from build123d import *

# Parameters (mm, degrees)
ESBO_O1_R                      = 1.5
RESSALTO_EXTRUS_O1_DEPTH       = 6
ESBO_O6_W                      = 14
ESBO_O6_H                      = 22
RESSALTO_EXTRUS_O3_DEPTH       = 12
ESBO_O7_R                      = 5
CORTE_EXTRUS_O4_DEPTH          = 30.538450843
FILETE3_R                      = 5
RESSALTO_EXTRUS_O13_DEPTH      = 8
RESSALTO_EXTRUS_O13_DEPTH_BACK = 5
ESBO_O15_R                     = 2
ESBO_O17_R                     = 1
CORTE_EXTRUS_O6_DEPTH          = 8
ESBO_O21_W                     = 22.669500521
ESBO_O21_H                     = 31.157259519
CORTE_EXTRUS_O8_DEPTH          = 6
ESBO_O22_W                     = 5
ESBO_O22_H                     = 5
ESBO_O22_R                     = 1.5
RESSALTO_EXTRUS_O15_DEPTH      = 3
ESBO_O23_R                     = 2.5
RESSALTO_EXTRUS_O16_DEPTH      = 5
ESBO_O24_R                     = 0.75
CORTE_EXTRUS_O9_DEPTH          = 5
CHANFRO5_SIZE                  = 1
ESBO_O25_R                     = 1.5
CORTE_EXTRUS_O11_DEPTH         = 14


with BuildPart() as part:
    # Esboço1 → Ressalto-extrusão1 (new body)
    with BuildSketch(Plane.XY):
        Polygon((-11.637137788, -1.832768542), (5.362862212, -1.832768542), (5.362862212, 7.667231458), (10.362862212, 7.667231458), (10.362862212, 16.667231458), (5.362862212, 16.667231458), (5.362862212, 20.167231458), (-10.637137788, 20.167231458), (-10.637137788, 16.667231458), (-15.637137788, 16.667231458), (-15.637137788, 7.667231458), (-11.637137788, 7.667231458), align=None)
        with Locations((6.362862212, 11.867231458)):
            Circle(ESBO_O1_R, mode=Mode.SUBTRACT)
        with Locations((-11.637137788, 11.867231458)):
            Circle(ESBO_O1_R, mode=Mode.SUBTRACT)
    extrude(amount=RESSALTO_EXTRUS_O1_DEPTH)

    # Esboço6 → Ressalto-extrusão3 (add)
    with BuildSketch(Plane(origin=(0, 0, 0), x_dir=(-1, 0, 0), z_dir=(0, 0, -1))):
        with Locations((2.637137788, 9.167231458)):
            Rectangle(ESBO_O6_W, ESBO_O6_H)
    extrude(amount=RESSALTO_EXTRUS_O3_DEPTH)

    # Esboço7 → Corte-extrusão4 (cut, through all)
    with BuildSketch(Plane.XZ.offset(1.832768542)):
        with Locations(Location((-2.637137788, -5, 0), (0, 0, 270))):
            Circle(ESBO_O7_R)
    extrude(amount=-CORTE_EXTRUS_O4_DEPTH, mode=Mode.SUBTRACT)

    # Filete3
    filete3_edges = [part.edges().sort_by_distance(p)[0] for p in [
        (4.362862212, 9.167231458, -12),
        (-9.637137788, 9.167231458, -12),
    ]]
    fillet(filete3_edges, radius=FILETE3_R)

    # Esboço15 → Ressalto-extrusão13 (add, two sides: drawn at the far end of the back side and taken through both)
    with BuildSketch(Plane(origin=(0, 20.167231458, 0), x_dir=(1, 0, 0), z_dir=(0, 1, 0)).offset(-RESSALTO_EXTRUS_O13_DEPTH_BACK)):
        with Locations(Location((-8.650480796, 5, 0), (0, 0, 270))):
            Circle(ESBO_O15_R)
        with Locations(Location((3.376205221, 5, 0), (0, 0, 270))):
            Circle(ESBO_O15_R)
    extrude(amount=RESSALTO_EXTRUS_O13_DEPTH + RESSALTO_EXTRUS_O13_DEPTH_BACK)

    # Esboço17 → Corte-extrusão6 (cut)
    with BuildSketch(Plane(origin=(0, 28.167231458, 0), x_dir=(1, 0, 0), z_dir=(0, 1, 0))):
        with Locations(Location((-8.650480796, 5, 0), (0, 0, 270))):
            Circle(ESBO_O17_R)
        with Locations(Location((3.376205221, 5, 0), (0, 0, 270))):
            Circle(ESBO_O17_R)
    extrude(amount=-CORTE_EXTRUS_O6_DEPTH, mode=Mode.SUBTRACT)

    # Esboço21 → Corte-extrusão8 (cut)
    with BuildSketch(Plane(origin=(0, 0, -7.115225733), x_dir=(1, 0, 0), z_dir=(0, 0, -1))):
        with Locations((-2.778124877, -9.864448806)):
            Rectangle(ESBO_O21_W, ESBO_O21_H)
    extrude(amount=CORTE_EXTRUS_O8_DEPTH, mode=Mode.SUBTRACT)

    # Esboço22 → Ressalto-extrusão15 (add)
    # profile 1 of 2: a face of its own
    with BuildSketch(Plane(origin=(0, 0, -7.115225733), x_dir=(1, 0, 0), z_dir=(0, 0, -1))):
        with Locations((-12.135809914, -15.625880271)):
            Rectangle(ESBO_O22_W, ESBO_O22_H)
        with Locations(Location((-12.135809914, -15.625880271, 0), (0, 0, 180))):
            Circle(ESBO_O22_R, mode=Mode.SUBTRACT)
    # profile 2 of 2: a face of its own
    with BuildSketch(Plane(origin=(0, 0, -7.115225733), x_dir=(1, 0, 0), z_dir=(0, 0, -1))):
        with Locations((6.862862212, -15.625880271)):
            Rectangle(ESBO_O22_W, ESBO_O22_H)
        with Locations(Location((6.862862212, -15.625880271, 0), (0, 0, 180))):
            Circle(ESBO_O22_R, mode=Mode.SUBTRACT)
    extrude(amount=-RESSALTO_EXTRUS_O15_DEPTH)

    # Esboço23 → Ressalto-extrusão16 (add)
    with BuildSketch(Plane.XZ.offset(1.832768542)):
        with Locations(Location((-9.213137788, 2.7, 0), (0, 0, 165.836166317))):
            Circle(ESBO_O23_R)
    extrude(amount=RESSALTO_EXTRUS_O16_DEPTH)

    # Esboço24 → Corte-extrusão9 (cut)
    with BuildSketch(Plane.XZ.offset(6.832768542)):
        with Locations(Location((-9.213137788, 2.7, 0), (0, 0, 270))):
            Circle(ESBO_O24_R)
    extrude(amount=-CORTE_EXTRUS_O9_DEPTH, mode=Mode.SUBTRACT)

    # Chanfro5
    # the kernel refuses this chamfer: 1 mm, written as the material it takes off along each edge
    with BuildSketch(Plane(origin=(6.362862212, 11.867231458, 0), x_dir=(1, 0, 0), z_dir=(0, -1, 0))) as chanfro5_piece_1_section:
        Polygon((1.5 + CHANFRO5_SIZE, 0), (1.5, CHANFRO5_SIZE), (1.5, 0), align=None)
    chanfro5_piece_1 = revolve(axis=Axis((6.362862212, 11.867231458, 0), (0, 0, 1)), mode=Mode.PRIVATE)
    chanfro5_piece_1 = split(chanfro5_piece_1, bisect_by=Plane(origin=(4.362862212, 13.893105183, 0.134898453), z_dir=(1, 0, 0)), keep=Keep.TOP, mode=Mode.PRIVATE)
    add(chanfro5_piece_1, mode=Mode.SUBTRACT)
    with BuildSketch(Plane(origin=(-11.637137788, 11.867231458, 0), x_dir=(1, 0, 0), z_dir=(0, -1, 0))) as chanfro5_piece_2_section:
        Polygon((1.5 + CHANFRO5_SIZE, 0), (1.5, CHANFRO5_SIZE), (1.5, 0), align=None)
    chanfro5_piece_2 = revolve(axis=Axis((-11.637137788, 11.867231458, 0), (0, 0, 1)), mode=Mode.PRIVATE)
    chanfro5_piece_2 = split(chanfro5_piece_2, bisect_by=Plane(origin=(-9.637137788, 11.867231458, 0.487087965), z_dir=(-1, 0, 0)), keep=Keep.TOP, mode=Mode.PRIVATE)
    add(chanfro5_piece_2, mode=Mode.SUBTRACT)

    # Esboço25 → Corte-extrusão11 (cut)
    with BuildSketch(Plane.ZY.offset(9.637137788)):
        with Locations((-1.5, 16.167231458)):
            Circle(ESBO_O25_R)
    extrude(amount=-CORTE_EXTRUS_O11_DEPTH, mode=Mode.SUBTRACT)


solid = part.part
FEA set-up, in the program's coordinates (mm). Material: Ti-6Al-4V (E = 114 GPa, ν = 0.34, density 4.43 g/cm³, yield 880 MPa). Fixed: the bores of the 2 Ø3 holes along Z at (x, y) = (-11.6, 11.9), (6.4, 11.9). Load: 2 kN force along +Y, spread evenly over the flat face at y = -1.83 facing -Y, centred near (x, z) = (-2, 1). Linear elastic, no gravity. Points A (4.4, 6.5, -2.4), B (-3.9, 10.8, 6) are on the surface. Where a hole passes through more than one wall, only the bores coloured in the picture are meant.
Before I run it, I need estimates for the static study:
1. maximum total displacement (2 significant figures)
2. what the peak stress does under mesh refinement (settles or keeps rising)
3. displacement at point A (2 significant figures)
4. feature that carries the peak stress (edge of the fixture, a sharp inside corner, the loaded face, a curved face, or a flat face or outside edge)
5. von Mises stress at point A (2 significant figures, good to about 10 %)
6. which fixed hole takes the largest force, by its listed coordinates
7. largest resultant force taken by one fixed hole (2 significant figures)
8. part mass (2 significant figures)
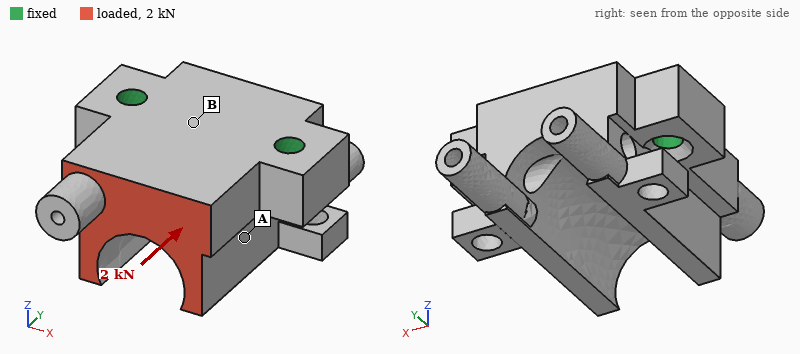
11 µm
keeps rising
5.4 µm
edge of the fixture
19 MPa
(6.4, 11.9)
1.1 kN
17 g
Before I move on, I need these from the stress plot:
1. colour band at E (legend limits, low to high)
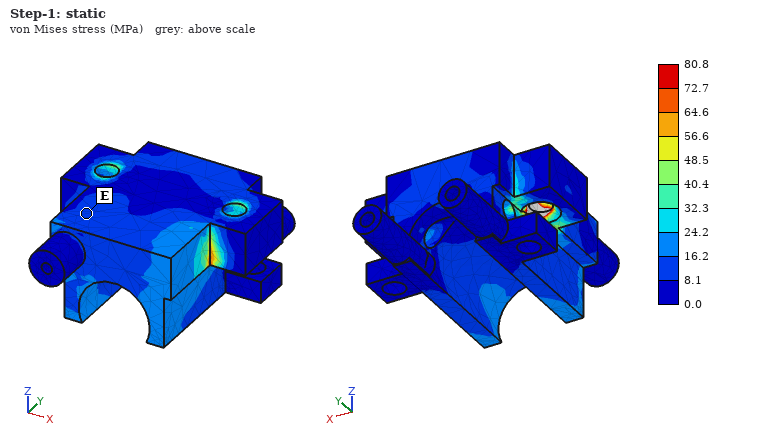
8.1 to 16.2 MPa
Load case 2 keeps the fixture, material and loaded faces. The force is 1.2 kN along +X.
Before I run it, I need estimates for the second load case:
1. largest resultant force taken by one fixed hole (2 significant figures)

1.1 kN
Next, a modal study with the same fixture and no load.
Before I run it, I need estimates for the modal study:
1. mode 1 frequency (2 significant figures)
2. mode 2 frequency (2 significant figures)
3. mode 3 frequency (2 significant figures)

14 kHz
16 kHz
16 kHz
